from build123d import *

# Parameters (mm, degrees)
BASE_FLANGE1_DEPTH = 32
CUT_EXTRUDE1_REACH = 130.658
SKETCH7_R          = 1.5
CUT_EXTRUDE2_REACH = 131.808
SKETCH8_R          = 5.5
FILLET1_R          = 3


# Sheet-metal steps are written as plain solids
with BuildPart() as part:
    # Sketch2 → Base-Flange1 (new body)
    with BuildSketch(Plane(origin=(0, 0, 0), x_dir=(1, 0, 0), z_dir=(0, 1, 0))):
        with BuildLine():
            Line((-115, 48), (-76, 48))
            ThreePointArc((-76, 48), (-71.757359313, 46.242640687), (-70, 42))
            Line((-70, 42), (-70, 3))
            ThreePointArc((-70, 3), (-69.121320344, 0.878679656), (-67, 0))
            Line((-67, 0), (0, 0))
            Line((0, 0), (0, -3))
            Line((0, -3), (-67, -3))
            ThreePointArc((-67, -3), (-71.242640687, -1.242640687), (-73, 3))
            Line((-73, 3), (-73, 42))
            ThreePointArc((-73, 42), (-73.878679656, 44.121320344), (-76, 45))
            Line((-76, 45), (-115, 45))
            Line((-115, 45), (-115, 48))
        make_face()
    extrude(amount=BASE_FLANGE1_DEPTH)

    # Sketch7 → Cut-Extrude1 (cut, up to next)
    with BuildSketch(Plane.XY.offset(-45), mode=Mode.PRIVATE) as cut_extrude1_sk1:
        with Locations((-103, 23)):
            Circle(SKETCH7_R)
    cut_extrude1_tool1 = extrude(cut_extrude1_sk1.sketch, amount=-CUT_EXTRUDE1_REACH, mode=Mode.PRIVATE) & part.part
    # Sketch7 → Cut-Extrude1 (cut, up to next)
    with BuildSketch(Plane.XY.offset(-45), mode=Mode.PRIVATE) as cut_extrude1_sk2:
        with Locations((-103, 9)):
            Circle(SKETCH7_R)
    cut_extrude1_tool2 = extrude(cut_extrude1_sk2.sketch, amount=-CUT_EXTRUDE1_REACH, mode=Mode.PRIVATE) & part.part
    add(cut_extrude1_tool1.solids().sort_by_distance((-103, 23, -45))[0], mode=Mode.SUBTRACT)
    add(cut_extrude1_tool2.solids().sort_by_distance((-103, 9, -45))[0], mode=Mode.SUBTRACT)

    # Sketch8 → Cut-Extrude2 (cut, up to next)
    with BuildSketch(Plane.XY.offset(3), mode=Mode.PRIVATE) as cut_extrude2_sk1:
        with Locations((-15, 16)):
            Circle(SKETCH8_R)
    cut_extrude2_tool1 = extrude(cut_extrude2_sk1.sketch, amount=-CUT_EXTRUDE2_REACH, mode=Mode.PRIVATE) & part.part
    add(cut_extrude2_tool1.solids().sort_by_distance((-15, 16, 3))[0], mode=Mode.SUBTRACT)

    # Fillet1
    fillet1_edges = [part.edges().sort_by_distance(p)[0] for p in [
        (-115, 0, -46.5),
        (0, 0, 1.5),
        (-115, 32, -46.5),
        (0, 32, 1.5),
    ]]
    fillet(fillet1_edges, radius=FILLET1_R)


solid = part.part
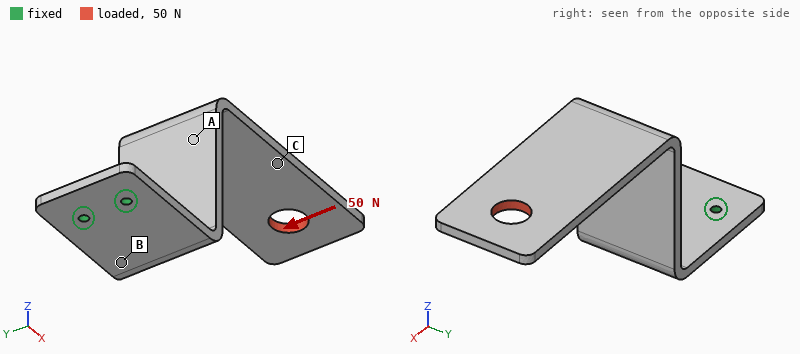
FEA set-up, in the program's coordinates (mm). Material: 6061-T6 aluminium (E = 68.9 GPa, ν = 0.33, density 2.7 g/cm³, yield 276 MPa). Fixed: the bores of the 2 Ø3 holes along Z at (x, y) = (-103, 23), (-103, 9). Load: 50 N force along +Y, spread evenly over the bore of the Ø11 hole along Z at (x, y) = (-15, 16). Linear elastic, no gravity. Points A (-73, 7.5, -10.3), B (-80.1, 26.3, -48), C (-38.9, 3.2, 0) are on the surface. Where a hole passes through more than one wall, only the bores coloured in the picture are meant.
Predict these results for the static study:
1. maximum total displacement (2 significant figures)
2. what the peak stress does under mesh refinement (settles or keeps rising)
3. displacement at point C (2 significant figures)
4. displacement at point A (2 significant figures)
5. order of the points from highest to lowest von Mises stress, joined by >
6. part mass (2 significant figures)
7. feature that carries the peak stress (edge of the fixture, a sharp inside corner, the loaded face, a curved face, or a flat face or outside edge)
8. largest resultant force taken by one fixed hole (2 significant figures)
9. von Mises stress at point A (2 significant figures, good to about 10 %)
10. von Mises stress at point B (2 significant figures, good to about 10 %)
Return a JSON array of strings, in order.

["1.3 mm", "keeps rising", "0.76 mm", "0.21 mm", "A > B > C", "40 g", "edge of the fixture", "310 N", "45 MPa", "26 MPa"]
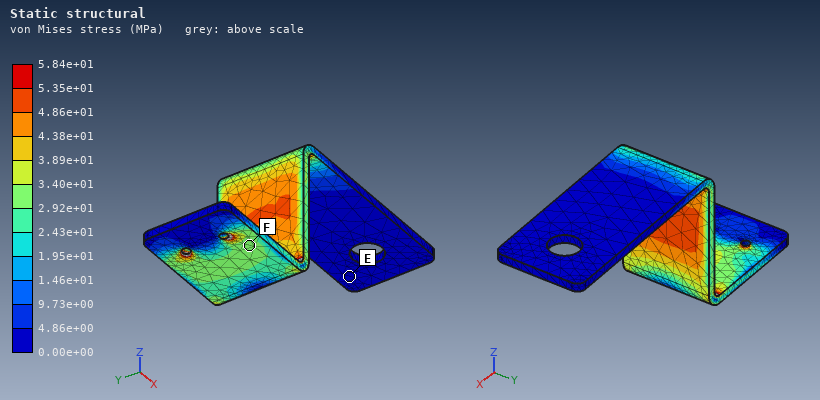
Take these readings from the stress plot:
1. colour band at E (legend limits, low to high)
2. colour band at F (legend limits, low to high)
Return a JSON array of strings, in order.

["0.00e+00 to 4.86e+00 MPa", "2.92e+01 to 3.40e+01 MPa"]
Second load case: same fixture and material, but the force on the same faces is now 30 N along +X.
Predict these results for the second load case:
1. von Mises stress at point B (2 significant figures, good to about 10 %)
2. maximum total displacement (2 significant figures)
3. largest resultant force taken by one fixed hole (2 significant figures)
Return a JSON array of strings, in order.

["28 MPa", "1.3 mm", "16 N"]
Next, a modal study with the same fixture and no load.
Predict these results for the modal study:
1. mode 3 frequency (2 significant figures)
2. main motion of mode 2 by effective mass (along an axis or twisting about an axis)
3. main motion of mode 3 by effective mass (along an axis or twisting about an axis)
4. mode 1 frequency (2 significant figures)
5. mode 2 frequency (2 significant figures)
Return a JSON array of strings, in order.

["590 Hz", "along Y", "along X", "160 Hz", "320 Hz"]
